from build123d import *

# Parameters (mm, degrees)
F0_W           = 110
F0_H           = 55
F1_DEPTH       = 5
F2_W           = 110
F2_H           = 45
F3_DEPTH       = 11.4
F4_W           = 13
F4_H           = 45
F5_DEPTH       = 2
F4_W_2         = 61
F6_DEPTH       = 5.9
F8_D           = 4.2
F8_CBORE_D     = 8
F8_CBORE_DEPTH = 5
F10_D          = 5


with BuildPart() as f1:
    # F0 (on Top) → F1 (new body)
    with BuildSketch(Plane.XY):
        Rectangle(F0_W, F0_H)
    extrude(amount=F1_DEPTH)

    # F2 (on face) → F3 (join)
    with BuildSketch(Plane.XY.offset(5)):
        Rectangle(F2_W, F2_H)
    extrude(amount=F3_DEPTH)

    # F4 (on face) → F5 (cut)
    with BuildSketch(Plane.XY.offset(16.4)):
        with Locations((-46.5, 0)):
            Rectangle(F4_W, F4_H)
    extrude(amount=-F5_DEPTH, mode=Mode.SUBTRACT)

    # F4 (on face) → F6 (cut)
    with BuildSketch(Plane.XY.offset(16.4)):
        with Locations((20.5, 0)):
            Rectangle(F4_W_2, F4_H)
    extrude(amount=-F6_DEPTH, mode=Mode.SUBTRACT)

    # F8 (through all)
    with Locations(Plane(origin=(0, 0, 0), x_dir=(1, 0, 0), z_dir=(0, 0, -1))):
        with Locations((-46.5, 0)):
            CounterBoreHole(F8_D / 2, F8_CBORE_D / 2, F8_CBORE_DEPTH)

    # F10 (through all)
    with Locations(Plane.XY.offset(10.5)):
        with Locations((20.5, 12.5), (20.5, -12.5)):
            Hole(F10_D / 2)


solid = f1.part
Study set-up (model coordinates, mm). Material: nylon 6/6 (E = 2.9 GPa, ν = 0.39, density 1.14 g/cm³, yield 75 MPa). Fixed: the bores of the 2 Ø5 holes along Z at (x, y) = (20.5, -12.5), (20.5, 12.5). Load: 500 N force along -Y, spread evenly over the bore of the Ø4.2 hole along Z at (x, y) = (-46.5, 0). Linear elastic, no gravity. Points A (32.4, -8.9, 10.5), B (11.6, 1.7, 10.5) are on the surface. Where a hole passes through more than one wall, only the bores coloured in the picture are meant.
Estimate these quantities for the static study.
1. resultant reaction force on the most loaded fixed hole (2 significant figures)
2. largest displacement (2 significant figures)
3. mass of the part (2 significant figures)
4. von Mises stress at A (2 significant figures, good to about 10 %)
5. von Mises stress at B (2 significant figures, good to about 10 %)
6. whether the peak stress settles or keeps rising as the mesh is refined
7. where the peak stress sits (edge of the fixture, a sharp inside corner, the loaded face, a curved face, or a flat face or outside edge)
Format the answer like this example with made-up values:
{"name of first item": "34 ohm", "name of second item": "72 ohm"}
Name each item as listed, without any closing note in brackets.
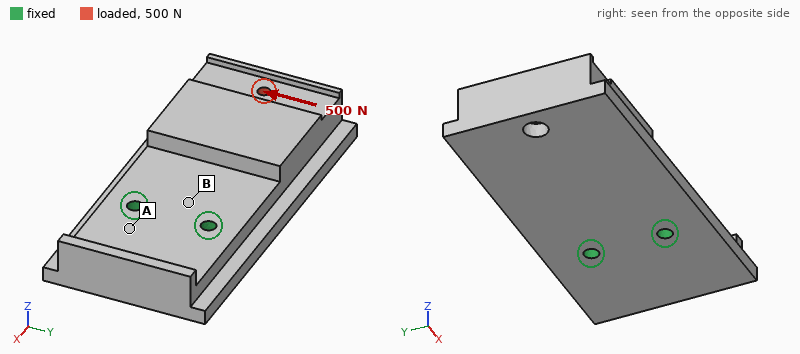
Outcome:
{"resultant reaction force on the most loaded fixed hole": "1.2 kN", "largest displacement": "0.36 mm", "mass of the part": "78 g", "von Mises stress at A": "1.7 MPa", "von Mises stress at B": "4.6 MPa", "whether the peak stress settles or keeps rising as the mesh is refined": "keeps rising", "where the peak stress sits": "edge of the fixture"}
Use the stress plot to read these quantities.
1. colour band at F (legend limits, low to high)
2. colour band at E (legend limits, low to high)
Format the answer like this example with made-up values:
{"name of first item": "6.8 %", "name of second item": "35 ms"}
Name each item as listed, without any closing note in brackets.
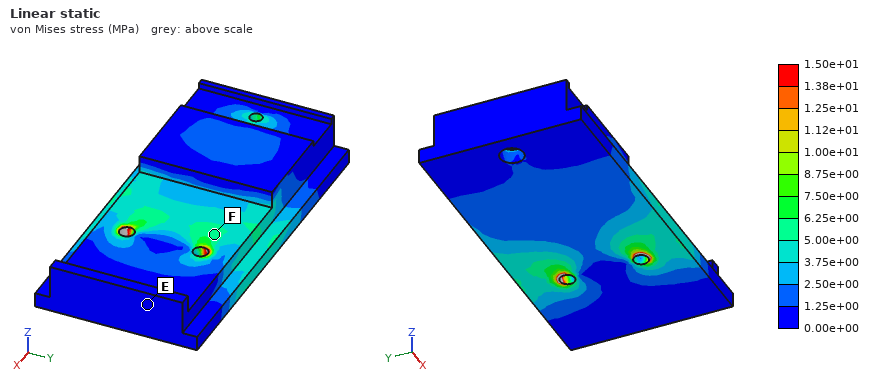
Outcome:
{"colour band at F": "5.00e+00 to 6.25e+00 MPa", "colour band at E": "0.00e+00 to 1.25e+00 MPa"}
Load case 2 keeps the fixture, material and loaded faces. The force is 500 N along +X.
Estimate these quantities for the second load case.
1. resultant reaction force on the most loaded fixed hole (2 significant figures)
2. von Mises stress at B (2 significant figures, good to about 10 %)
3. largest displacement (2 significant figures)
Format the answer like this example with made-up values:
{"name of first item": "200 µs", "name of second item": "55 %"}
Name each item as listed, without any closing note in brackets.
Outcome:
{"resultant reaction force on the most loaded fixed hole": "250 N", "von Mises stress at B": "2.8 MPa", "largest displacement": "0.37 mm"}
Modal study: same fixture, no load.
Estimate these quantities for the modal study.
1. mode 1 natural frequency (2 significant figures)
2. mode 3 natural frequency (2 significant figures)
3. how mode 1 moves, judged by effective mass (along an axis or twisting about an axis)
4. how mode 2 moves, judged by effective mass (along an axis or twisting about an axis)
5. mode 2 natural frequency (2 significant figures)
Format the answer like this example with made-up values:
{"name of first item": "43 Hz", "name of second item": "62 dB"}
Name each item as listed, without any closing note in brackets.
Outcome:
{"mode 1 natural frequency": "400 Hz", "mode 3 natural frequency": "1400 Hz", "how mode 1 moves, judged by effective mass": "along Z", "how mode 2 moves, judged by effective mass": "along Y", "mode 2 natural frequency": "1300 Hz"}
